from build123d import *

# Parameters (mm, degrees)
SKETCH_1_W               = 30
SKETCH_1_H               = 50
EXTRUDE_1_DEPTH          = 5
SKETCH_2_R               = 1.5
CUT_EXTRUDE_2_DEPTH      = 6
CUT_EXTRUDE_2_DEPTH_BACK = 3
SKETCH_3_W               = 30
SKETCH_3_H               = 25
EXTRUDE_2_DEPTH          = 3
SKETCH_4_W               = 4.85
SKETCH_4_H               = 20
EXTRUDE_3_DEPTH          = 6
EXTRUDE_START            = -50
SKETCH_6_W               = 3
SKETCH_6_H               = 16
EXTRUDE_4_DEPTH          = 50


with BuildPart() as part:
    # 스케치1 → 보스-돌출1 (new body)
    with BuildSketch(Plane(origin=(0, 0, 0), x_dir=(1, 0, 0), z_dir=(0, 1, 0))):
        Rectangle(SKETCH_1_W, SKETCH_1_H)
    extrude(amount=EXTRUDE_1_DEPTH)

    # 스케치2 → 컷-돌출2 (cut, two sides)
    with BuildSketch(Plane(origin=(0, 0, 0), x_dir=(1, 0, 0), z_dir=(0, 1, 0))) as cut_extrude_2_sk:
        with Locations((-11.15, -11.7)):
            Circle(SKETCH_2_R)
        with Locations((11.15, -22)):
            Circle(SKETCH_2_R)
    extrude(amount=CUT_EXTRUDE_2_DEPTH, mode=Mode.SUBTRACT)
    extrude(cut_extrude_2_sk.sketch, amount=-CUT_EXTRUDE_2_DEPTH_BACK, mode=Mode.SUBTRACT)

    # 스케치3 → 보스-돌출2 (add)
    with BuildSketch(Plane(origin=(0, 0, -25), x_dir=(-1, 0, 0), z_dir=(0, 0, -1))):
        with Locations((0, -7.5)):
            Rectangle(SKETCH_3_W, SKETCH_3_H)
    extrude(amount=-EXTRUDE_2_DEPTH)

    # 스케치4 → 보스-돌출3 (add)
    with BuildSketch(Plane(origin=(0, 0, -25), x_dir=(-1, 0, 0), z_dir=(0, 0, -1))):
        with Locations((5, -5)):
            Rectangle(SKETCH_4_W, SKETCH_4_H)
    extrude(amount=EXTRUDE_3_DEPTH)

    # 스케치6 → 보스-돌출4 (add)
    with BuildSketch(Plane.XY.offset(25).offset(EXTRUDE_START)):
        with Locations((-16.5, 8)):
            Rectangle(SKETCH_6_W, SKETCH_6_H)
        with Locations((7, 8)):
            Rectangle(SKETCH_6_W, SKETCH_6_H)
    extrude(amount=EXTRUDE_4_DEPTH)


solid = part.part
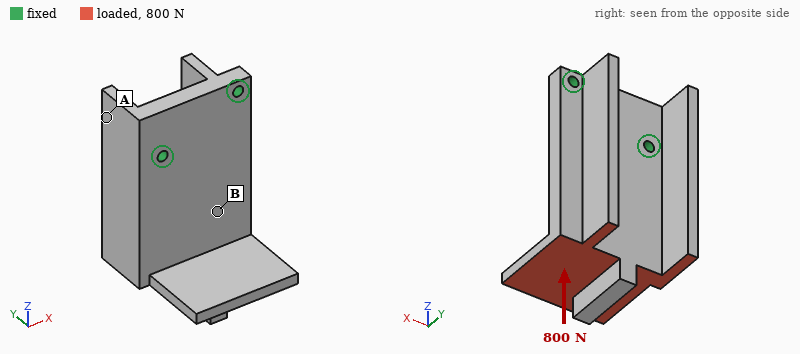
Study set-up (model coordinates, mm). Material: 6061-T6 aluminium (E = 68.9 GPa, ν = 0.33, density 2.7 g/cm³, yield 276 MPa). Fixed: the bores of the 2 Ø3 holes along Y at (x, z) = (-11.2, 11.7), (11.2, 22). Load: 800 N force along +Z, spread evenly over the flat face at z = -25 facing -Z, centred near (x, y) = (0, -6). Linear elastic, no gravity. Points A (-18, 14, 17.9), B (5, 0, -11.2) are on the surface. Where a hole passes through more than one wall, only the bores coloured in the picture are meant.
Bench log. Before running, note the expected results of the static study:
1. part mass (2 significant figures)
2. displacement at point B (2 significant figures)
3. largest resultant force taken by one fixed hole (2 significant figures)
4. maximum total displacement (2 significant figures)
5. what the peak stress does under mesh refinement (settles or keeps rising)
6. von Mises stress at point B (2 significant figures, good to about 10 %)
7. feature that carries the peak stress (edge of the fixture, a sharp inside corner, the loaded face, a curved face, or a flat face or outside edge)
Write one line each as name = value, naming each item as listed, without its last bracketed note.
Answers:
part mass = 37 g
displacement at point B = 0.043 mm
largest resultant force taken by one fixed hole = 430 N
maximum total displacement = 0.21 mm
what the peak stress does under mesh refinement = keeps rising
von Mises stress at point B = 20 MPa
feature that carries the peak stress = edge of the fixture
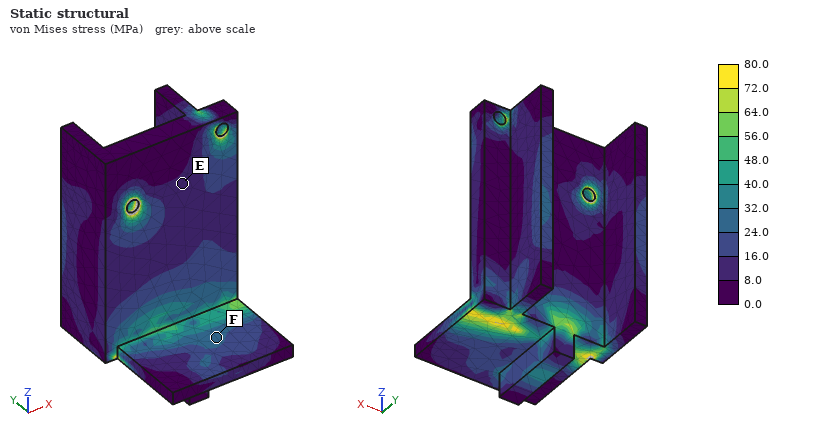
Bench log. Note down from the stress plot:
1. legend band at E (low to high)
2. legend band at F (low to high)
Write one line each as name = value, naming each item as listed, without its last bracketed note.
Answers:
legend band at E = 8.0 to 16.0 MPa
legend band at F = 24.0 to 32.0 MPa
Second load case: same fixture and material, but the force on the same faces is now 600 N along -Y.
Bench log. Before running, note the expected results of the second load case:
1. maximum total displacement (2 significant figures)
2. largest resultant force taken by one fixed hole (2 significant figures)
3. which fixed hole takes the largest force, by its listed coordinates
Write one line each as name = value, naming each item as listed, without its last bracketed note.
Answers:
maximum total displacement = 0.32 mm
largest resultant force taken by one fixed hole = 660 N
which fixed hole takes the largest force, by its listed coordinates = (-11.2, 11.7)
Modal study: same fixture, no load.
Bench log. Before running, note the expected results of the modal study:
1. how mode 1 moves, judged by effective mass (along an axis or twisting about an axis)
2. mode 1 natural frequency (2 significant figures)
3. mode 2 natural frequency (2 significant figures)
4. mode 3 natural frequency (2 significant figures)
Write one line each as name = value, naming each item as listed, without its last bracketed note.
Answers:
how mode 1 moves, judged by effective mass = along Y
mode 1 natural frequency = 2100 Hz
mode 2 natural frequency = 3700 Hz
mode 3 natural frequency = 6100 Hz
